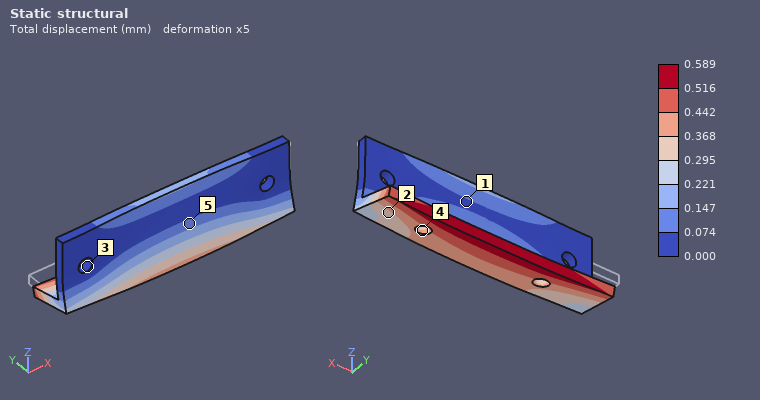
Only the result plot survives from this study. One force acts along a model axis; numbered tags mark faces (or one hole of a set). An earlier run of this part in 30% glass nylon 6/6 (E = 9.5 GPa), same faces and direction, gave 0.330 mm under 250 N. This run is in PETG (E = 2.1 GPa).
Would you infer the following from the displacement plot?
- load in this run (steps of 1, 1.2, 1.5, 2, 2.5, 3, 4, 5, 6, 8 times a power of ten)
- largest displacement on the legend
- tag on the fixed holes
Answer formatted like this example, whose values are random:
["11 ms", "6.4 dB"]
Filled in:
["100 N", "0.589 mm", "3"]
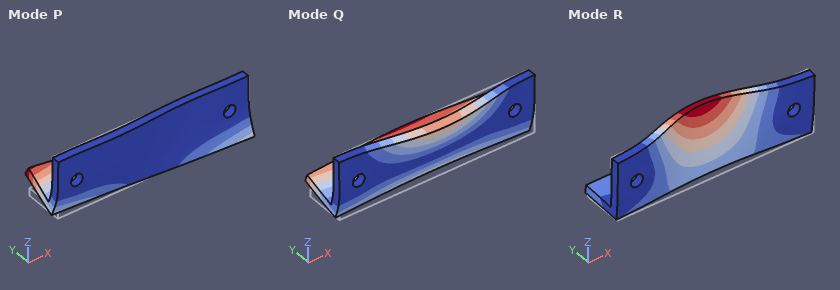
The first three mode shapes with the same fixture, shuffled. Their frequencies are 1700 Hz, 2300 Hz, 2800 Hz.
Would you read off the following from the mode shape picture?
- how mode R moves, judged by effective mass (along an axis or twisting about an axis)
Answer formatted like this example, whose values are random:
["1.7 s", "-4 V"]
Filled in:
["along Y"]
